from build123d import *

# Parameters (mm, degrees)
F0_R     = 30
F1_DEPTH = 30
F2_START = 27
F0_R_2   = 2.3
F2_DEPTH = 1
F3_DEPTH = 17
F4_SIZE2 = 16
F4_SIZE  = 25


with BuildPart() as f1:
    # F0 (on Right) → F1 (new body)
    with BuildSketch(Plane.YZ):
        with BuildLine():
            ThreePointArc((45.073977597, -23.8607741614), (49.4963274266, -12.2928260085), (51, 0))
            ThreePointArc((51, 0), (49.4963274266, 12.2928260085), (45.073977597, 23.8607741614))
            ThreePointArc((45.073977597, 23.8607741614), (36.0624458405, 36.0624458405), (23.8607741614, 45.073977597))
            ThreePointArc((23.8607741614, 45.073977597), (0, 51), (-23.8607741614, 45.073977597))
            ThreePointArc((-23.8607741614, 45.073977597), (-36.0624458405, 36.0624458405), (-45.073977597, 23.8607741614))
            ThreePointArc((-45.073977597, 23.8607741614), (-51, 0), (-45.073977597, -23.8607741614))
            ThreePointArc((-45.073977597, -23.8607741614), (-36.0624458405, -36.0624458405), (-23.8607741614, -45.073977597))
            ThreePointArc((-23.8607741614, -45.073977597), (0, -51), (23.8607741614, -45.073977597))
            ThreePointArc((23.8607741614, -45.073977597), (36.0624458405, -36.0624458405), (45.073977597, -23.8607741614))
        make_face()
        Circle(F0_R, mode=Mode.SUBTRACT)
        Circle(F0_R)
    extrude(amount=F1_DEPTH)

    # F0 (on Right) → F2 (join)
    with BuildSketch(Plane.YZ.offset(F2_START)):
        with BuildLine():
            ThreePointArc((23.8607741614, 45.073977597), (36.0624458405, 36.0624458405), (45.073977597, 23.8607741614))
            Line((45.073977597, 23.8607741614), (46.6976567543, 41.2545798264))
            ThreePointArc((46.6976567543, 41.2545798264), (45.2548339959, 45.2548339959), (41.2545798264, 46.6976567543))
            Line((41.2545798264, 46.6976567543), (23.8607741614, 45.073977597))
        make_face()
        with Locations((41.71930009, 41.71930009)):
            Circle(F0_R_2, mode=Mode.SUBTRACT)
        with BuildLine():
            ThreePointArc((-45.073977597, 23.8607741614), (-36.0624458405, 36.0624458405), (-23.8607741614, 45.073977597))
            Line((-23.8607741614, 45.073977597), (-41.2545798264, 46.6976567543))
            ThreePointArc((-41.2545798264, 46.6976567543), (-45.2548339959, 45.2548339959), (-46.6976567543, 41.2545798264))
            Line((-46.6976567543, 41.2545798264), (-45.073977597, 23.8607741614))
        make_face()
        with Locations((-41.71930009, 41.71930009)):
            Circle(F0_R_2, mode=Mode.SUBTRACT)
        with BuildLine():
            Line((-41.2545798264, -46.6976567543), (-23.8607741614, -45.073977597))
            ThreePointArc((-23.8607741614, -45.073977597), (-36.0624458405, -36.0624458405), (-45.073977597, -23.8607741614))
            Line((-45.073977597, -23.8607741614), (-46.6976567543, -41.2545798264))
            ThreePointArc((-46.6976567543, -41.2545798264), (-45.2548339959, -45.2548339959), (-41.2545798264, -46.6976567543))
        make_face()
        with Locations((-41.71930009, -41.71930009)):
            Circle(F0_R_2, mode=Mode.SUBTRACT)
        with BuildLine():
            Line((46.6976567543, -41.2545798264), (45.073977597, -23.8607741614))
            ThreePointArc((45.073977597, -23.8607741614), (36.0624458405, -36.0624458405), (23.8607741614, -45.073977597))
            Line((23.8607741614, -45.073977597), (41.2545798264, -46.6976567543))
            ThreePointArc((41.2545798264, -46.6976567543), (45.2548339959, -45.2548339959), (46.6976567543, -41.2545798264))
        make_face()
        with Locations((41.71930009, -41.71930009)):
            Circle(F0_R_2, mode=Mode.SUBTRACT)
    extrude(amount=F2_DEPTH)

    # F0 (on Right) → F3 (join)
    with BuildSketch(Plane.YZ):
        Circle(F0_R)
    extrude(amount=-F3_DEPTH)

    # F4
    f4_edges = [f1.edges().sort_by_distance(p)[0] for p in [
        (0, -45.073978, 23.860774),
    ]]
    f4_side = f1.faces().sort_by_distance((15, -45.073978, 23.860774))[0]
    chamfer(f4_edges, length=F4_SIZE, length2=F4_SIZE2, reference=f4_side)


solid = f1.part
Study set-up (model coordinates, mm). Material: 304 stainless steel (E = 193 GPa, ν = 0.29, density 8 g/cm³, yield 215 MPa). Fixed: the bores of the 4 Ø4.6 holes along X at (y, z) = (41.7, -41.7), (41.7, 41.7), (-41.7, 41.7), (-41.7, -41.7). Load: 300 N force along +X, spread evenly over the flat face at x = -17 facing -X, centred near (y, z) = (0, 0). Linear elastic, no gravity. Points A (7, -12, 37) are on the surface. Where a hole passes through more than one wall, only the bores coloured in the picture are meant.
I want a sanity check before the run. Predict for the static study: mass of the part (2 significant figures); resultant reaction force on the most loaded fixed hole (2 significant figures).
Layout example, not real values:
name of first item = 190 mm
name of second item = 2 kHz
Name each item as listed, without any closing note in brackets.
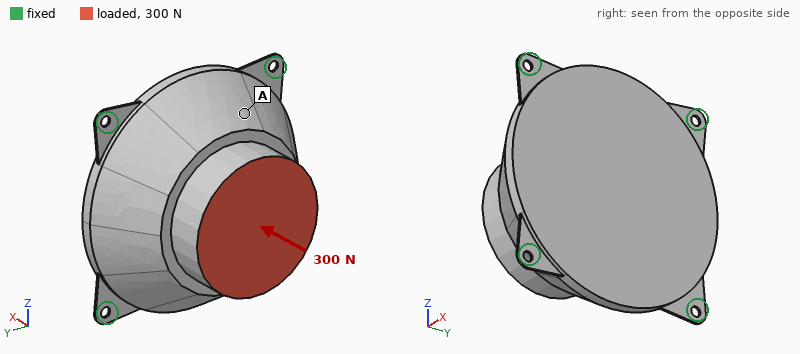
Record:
mass of the part = 1.9 kg
resultant reaction force on the most loaded fixed hole = 78 N
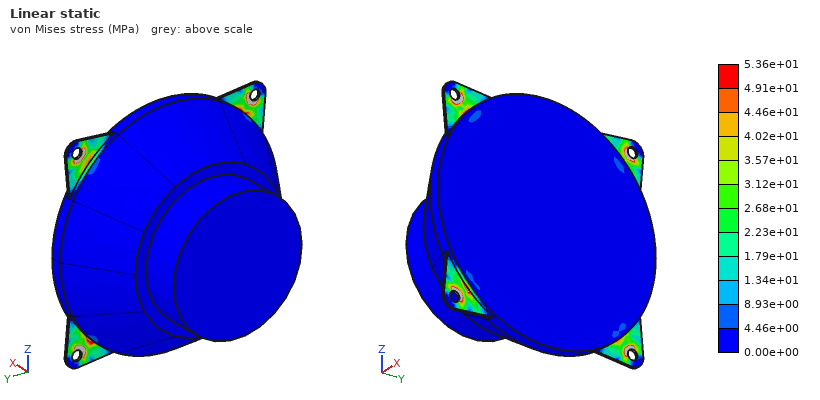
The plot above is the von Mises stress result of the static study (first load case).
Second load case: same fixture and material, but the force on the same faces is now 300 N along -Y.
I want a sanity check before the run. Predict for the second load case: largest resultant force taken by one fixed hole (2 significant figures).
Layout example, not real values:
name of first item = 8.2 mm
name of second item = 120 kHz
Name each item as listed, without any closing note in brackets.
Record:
largest resultant force taken by one fixed hole = 120 N
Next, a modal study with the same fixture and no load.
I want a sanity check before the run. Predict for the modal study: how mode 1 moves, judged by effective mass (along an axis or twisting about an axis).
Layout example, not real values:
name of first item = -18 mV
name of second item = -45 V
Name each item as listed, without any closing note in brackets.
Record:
how mode 1 moves, judged by effective mass = along X
